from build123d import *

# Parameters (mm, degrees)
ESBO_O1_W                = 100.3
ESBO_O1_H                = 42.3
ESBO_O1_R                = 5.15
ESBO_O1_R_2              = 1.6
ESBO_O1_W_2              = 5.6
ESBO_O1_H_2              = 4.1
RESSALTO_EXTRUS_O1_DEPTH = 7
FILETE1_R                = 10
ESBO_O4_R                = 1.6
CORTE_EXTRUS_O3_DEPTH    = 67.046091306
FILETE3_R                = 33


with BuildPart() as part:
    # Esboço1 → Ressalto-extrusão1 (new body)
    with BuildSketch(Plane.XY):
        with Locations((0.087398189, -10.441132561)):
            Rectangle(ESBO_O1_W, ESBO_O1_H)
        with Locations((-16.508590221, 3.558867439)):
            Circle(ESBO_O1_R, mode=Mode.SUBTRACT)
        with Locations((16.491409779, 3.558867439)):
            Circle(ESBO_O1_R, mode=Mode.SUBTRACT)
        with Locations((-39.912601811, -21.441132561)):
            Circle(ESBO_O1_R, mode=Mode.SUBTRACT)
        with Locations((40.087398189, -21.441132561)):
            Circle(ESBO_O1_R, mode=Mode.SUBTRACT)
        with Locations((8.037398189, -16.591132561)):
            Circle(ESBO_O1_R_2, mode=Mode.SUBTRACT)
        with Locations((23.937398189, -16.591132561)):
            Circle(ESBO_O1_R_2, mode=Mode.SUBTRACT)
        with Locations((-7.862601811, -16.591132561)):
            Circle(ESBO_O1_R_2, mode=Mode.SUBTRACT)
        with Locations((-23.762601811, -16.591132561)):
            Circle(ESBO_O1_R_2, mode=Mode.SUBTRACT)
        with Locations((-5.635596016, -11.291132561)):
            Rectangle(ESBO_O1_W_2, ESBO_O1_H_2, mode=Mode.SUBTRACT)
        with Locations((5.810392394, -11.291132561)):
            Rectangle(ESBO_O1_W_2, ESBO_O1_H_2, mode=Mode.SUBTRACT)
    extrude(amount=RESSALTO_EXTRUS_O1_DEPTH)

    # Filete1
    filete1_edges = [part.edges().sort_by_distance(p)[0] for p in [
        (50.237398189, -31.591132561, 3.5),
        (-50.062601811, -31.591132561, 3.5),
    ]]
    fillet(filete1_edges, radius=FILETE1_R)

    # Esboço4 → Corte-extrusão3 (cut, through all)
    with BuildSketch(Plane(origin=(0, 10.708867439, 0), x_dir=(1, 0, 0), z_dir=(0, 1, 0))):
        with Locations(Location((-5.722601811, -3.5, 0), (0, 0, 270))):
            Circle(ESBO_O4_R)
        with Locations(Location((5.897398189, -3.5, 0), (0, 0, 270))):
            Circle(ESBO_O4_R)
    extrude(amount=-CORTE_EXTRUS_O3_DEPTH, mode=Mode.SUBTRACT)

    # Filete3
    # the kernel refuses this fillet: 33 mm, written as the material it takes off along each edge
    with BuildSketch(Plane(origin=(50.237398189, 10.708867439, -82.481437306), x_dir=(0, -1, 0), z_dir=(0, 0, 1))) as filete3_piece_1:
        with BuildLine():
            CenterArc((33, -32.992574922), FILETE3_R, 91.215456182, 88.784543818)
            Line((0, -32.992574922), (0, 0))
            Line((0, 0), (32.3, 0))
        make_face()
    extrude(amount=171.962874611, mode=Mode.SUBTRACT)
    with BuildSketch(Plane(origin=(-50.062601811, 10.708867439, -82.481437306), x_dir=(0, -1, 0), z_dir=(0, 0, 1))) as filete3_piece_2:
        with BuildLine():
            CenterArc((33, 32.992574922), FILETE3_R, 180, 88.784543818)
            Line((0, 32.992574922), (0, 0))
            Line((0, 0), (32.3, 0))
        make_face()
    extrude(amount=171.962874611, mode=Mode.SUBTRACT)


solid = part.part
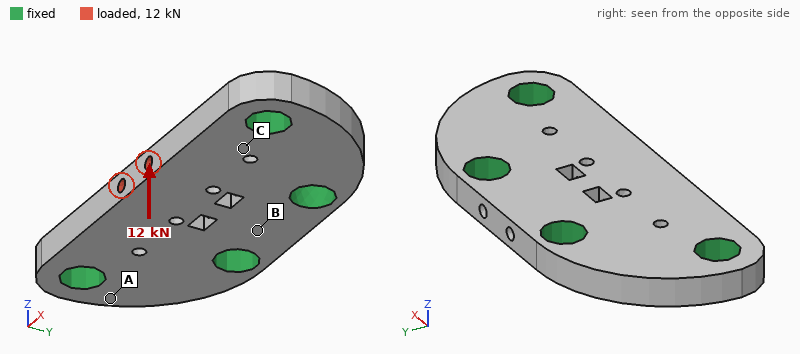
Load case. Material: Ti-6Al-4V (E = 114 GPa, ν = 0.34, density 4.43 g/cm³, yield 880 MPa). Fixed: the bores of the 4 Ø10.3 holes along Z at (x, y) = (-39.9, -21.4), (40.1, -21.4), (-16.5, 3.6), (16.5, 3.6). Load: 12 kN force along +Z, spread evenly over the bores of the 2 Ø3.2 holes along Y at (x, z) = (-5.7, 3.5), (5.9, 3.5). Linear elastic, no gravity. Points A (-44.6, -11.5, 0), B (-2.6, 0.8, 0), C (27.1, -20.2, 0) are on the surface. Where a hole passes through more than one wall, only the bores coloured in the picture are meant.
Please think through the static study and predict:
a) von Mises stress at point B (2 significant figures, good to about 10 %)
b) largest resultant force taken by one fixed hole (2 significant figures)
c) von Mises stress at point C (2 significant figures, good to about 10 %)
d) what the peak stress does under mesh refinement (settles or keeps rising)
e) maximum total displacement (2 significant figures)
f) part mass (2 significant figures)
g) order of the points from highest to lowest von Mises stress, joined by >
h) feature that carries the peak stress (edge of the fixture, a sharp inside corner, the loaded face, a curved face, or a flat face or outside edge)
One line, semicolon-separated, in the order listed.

120 MPa; 3.3 kN; 200 MPa; keeps rising; 0.28 mm; 100 g; C > B > A; a sharp inside corner
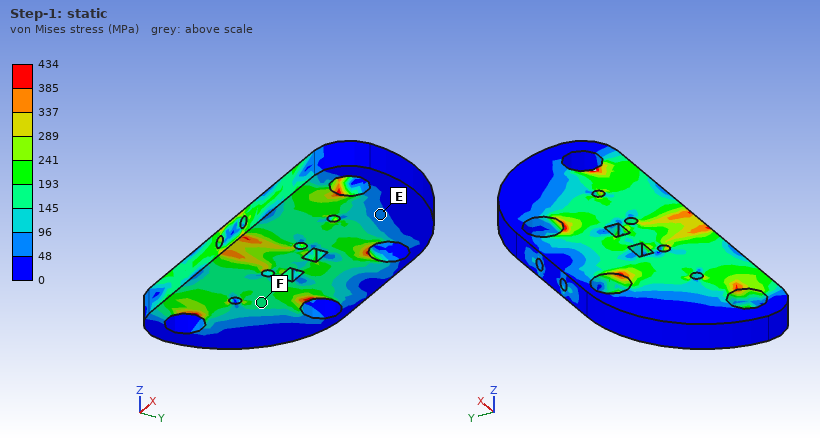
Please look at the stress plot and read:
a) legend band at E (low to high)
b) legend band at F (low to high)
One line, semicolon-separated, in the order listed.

48 to 96 MPa; 145 to 193 MPa
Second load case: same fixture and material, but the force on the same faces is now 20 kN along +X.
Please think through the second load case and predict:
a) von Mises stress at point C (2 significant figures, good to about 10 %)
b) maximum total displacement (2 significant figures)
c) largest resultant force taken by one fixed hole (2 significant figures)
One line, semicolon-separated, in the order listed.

69 MPa; 20 µm; 7.1 kN
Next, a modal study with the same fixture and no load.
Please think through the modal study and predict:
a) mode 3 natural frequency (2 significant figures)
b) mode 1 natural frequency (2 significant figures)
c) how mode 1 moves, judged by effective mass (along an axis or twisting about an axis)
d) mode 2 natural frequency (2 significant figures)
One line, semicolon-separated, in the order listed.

25 kHz; 9600 Hz; along Z; 19 kHz
